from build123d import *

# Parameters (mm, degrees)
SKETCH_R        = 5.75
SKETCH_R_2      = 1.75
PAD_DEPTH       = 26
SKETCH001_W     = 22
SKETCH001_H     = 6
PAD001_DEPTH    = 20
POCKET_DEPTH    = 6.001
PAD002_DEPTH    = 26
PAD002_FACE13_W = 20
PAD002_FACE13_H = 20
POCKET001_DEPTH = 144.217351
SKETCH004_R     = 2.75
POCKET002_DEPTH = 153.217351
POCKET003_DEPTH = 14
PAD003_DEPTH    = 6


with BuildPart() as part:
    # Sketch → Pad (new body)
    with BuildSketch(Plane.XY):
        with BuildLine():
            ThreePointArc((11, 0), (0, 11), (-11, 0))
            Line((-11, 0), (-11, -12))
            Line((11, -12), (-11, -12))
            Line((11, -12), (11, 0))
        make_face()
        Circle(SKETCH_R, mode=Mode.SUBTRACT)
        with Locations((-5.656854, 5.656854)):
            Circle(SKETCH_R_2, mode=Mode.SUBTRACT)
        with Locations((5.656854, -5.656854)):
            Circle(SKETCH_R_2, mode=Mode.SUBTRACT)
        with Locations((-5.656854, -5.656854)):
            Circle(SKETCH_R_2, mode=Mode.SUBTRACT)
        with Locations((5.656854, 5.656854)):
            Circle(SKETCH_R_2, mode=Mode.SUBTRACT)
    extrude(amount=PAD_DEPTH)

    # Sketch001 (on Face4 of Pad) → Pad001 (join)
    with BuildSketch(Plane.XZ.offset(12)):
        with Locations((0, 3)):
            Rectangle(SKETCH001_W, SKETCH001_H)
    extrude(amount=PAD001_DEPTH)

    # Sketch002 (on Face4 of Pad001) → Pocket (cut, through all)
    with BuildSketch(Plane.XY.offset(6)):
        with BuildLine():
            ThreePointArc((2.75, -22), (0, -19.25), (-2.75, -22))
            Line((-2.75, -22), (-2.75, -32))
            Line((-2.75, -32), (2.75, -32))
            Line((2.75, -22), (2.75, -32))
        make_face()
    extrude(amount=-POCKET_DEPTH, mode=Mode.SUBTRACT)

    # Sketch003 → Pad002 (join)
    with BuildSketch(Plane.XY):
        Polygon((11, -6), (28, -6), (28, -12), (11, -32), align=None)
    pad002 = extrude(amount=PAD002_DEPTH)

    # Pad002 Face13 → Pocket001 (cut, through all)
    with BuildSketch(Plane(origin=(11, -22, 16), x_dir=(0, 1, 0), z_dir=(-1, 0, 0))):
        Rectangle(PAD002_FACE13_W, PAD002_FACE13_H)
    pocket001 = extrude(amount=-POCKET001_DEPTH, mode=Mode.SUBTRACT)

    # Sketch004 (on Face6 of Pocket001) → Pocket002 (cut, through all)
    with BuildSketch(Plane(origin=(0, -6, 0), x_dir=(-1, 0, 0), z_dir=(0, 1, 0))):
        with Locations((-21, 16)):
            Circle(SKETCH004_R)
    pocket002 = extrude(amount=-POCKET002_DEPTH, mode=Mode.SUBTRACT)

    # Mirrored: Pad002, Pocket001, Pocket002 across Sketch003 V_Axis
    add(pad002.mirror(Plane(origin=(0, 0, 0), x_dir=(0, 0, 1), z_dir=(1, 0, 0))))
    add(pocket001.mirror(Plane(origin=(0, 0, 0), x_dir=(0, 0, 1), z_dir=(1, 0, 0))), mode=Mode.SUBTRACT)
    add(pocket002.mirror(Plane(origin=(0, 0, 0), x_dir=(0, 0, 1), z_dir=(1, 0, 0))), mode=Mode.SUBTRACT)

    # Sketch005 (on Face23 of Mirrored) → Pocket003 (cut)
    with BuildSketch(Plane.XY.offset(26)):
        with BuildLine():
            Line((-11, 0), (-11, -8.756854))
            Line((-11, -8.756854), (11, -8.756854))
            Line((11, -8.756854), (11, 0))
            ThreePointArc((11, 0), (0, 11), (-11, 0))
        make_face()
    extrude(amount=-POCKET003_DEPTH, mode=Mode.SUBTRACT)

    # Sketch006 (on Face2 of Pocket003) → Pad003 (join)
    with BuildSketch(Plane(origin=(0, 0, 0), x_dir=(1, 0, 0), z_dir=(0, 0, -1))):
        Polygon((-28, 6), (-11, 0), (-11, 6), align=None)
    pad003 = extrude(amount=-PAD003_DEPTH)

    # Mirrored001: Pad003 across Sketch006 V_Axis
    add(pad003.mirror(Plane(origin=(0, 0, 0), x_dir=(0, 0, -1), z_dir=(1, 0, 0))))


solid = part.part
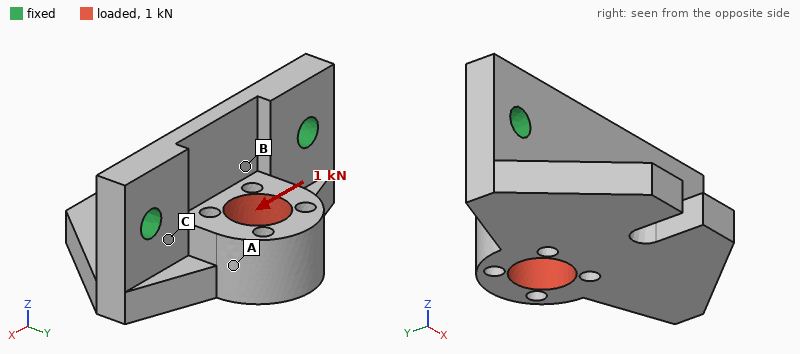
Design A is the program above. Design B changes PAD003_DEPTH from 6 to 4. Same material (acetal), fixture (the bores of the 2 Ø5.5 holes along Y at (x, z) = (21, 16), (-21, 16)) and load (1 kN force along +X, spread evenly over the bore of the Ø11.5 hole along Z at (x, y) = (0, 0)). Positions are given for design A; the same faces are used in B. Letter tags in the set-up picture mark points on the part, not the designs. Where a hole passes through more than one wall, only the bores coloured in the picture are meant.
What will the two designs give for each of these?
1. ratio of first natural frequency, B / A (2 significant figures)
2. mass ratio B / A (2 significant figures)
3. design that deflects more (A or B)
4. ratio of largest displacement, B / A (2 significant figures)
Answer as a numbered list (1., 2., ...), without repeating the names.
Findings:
1. 1.00
2. 0.99
3. B
4. 1.1
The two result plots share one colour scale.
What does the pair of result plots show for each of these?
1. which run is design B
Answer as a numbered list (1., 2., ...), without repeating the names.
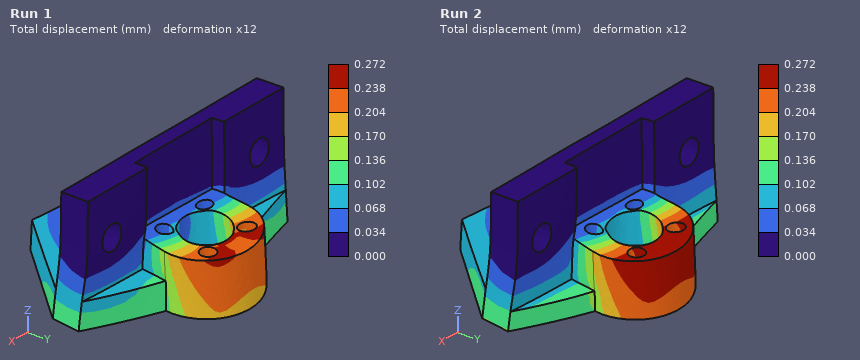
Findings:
1. Run 2
